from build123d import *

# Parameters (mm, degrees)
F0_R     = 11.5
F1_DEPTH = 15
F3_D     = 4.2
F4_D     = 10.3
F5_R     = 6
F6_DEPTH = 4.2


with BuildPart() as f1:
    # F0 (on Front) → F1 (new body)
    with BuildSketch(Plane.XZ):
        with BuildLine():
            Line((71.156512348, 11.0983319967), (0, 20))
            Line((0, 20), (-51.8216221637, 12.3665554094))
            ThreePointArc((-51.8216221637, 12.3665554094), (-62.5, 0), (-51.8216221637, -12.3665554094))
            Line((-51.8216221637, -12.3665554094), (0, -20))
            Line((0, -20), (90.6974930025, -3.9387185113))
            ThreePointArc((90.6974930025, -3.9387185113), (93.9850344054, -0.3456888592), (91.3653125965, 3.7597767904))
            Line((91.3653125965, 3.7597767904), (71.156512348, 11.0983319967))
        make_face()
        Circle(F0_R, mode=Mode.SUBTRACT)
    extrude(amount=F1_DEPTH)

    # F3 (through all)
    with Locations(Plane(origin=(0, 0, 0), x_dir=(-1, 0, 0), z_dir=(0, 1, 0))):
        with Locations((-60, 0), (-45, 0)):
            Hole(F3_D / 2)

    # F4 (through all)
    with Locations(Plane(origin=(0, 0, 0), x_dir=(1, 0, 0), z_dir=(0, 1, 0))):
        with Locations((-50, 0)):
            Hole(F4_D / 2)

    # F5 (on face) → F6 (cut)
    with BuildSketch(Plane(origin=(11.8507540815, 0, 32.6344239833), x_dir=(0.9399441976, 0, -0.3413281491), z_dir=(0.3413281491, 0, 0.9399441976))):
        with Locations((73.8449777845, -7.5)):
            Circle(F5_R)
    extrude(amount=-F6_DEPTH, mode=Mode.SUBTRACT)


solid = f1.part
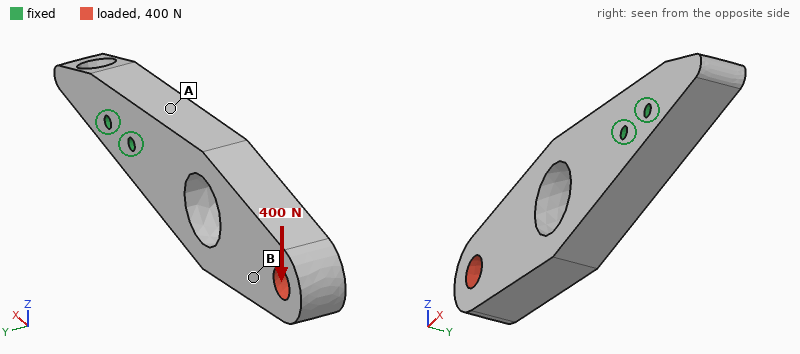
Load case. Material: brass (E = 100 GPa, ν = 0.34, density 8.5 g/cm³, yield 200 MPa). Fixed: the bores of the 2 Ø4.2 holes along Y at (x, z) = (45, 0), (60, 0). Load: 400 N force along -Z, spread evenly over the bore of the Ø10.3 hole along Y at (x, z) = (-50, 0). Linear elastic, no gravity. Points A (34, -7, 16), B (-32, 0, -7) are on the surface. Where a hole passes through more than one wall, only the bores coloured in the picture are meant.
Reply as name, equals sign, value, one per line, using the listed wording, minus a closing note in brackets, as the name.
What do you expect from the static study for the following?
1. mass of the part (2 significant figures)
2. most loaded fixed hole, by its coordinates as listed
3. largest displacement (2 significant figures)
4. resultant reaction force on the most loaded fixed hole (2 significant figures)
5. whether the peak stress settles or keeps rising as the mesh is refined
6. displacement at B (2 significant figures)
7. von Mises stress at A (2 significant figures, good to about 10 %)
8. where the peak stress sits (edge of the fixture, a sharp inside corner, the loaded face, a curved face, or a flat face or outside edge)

mass of the part = 470 g
most loaded fixed hole, by its coordinates as listed = (45, 0)
largest displacement = 71 µm
resultant reaction force on the most loaded fixed hole = 2.3 kN
whether the peak stress settles or keeps rising as the mesh is refined = keeps rising
displacement at B = 49 µm
von Mises stress at A = 16 MPa
where the peak stress sits = edge of the fixture
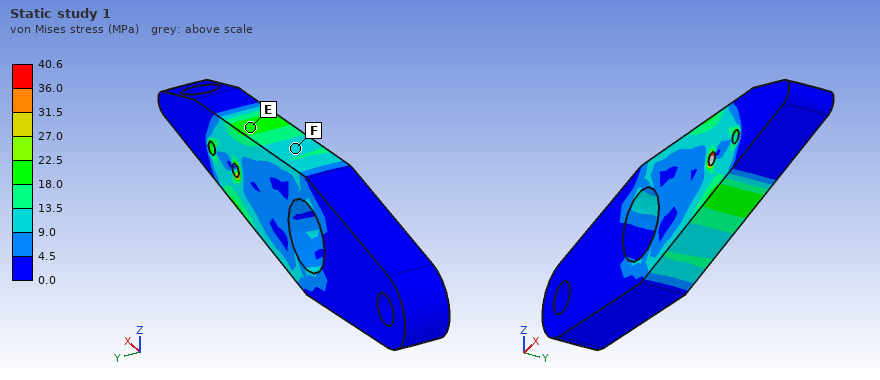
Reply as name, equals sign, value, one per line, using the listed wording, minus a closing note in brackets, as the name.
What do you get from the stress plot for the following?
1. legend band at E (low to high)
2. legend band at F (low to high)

legend band at E = 18.0 to 22.5 MPa
legend band at F = 9.0 to 13.5 MPa
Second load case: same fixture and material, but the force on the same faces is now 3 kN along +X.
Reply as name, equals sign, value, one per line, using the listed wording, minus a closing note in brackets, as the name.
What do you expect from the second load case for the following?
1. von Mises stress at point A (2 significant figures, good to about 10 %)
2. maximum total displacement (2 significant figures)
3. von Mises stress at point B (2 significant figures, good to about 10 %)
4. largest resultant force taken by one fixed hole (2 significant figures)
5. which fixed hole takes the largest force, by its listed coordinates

von Mises stress at point A = 5.6 MPa
maximum total displacement = 12 µm
von Mises stress at point B = 6.2 MPa
largest resultant force taken by one fixed hole = 2.3 kN
which fixed hole takes the largest force, by its listed coordinates = (45, 0)
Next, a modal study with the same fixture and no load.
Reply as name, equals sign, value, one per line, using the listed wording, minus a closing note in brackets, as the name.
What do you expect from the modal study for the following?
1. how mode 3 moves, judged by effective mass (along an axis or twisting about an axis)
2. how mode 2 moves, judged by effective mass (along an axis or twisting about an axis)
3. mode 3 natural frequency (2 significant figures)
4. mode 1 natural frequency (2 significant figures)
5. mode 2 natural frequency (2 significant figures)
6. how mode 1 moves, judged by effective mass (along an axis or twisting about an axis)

how mode 3 moves, judged by effective mass = twisting about X
how mode 2 moves, judged by effective mass = along Z
mode 3 natural frequency = 3300 Hz
mode 1 natural frequency = 710 Hz
mode 2 natural frequency = 1100 Hz
how mode 1 moves, judged by effective mass = along Y
